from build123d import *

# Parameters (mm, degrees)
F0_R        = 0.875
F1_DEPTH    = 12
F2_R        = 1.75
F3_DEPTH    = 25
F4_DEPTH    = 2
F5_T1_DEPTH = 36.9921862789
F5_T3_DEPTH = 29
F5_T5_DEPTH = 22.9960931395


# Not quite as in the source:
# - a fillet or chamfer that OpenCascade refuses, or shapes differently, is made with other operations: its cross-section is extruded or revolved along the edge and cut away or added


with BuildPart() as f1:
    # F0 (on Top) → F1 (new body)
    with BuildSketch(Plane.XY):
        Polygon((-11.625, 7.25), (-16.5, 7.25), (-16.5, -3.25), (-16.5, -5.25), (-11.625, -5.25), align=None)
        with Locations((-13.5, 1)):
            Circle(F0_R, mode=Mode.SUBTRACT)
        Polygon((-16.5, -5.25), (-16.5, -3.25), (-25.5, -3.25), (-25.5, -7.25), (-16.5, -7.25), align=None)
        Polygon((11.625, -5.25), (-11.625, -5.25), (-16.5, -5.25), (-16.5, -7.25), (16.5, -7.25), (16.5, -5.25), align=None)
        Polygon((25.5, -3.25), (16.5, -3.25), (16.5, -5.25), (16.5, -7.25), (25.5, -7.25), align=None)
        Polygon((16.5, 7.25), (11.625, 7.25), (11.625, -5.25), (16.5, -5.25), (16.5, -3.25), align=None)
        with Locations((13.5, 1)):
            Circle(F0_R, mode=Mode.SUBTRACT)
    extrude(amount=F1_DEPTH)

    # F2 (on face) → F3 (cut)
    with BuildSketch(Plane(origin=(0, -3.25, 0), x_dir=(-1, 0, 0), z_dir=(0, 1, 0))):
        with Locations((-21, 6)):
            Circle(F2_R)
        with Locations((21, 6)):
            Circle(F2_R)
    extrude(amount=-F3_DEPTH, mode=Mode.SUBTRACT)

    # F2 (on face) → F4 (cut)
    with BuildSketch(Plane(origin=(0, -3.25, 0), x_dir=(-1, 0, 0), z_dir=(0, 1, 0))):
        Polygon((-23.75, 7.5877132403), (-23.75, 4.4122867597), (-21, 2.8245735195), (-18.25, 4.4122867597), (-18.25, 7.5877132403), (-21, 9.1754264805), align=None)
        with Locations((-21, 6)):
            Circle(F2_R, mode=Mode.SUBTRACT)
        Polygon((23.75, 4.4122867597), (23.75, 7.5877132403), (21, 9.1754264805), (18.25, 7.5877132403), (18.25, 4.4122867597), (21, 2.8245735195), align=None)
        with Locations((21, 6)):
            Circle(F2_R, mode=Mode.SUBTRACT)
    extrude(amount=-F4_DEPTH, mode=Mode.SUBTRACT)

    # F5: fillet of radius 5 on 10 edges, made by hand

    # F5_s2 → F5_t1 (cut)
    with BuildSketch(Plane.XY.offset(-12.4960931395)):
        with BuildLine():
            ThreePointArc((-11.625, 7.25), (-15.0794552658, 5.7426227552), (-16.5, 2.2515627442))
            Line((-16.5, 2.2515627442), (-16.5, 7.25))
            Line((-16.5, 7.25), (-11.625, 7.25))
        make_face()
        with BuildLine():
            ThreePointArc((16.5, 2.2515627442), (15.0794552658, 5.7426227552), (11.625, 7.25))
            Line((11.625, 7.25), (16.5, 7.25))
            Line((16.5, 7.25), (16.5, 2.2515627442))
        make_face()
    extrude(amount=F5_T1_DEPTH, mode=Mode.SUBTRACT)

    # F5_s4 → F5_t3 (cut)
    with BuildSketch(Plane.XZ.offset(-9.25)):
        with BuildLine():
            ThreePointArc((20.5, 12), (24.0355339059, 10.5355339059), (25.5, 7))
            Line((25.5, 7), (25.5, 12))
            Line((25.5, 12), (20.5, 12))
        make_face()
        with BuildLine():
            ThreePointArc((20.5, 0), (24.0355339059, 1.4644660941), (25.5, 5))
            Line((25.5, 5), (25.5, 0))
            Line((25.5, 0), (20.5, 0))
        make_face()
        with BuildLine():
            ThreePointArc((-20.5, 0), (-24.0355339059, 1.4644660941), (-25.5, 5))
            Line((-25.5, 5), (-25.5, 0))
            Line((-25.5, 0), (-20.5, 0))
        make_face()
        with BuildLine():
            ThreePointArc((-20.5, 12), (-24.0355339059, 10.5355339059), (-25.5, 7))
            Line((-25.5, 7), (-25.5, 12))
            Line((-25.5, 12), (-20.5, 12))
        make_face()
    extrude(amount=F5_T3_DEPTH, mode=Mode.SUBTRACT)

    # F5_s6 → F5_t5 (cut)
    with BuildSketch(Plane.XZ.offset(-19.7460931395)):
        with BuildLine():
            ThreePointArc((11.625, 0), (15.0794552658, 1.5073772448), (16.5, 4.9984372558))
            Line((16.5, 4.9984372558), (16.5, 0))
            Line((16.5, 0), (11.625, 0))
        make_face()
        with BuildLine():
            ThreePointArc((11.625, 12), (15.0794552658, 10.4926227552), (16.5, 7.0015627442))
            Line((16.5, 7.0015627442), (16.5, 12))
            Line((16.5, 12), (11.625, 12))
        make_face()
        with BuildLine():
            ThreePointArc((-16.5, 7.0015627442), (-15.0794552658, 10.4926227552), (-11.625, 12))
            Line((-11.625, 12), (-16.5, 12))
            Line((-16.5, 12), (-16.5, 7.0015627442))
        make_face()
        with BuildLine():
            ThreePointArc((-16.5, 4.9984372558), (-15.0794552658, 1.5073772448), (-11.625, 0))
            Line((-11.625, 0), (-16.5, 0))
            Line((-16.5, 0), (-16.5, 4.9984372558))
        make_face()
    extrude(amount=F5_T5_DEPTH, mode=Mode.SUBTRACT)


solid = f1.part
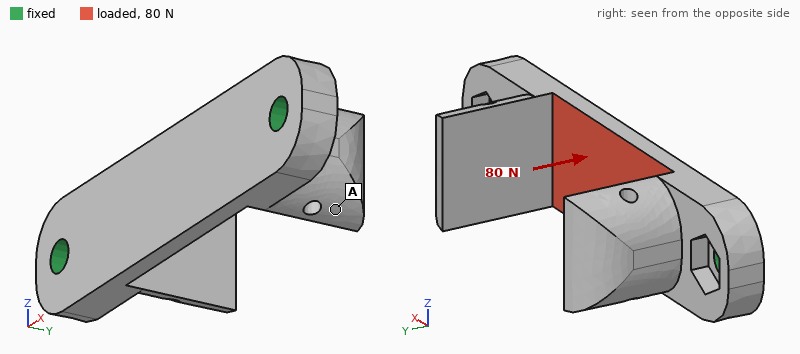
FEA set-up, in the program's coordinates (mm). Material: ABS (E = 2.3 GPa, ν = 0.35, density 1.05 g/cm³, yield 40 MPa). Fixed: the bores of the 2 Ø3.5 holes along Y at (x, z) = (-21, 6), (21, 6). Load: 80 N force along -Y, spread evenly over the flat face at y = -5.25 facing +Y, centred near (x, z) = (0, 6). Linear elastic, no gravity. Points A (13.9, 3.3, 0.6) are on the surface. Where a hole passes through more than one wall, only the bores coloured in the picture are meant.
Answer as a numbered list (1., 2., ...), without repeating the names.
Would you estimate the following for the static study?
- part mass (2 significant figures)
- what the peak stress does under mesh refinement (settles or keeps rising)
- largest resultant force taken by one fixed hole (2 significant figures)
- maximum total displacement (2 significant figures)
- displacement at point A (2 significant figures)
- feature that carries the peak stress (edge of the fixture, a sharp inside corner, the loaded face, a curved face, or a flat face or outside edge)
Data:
1. 2.7 g
2. keeps rising
3. 48 N
4. 0.59 mm
5. 0.31 mm
6. edge of the fixture
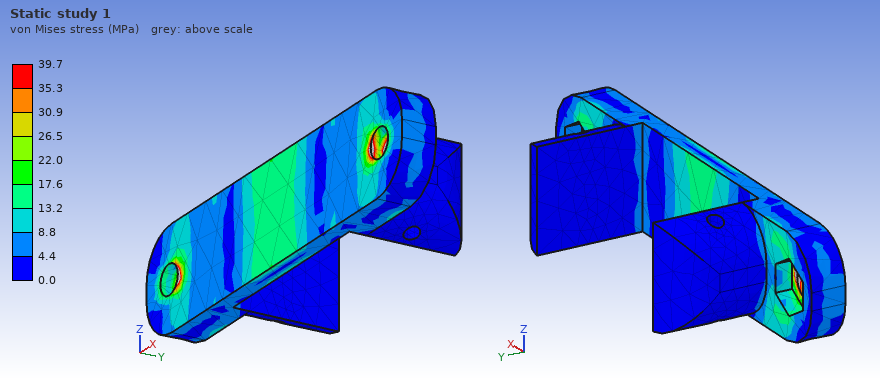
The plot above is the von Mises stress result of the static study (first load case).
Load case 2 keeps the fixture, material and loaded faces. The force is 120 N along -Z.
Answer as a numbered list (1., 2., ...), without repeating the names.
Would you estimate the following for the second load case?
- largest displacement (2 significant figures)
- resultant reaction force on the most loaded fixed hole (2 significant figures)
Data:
1. 0.16 mm
2. 60 N
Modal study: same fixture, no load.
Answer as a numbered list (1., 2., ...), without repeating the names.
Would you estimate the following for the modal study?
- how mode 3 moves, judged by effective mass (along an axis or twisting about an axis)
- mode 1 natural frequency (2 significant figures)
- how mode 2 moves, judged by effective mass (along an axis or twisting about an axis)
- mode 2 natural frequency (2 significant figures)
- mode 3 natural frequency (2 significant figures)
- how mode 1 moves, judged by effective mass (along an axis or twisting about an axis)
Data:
1. along Z
2. 2000 Hz
3. along X
4. 2900 Hz
5. 3100 Hz
6. along Y
